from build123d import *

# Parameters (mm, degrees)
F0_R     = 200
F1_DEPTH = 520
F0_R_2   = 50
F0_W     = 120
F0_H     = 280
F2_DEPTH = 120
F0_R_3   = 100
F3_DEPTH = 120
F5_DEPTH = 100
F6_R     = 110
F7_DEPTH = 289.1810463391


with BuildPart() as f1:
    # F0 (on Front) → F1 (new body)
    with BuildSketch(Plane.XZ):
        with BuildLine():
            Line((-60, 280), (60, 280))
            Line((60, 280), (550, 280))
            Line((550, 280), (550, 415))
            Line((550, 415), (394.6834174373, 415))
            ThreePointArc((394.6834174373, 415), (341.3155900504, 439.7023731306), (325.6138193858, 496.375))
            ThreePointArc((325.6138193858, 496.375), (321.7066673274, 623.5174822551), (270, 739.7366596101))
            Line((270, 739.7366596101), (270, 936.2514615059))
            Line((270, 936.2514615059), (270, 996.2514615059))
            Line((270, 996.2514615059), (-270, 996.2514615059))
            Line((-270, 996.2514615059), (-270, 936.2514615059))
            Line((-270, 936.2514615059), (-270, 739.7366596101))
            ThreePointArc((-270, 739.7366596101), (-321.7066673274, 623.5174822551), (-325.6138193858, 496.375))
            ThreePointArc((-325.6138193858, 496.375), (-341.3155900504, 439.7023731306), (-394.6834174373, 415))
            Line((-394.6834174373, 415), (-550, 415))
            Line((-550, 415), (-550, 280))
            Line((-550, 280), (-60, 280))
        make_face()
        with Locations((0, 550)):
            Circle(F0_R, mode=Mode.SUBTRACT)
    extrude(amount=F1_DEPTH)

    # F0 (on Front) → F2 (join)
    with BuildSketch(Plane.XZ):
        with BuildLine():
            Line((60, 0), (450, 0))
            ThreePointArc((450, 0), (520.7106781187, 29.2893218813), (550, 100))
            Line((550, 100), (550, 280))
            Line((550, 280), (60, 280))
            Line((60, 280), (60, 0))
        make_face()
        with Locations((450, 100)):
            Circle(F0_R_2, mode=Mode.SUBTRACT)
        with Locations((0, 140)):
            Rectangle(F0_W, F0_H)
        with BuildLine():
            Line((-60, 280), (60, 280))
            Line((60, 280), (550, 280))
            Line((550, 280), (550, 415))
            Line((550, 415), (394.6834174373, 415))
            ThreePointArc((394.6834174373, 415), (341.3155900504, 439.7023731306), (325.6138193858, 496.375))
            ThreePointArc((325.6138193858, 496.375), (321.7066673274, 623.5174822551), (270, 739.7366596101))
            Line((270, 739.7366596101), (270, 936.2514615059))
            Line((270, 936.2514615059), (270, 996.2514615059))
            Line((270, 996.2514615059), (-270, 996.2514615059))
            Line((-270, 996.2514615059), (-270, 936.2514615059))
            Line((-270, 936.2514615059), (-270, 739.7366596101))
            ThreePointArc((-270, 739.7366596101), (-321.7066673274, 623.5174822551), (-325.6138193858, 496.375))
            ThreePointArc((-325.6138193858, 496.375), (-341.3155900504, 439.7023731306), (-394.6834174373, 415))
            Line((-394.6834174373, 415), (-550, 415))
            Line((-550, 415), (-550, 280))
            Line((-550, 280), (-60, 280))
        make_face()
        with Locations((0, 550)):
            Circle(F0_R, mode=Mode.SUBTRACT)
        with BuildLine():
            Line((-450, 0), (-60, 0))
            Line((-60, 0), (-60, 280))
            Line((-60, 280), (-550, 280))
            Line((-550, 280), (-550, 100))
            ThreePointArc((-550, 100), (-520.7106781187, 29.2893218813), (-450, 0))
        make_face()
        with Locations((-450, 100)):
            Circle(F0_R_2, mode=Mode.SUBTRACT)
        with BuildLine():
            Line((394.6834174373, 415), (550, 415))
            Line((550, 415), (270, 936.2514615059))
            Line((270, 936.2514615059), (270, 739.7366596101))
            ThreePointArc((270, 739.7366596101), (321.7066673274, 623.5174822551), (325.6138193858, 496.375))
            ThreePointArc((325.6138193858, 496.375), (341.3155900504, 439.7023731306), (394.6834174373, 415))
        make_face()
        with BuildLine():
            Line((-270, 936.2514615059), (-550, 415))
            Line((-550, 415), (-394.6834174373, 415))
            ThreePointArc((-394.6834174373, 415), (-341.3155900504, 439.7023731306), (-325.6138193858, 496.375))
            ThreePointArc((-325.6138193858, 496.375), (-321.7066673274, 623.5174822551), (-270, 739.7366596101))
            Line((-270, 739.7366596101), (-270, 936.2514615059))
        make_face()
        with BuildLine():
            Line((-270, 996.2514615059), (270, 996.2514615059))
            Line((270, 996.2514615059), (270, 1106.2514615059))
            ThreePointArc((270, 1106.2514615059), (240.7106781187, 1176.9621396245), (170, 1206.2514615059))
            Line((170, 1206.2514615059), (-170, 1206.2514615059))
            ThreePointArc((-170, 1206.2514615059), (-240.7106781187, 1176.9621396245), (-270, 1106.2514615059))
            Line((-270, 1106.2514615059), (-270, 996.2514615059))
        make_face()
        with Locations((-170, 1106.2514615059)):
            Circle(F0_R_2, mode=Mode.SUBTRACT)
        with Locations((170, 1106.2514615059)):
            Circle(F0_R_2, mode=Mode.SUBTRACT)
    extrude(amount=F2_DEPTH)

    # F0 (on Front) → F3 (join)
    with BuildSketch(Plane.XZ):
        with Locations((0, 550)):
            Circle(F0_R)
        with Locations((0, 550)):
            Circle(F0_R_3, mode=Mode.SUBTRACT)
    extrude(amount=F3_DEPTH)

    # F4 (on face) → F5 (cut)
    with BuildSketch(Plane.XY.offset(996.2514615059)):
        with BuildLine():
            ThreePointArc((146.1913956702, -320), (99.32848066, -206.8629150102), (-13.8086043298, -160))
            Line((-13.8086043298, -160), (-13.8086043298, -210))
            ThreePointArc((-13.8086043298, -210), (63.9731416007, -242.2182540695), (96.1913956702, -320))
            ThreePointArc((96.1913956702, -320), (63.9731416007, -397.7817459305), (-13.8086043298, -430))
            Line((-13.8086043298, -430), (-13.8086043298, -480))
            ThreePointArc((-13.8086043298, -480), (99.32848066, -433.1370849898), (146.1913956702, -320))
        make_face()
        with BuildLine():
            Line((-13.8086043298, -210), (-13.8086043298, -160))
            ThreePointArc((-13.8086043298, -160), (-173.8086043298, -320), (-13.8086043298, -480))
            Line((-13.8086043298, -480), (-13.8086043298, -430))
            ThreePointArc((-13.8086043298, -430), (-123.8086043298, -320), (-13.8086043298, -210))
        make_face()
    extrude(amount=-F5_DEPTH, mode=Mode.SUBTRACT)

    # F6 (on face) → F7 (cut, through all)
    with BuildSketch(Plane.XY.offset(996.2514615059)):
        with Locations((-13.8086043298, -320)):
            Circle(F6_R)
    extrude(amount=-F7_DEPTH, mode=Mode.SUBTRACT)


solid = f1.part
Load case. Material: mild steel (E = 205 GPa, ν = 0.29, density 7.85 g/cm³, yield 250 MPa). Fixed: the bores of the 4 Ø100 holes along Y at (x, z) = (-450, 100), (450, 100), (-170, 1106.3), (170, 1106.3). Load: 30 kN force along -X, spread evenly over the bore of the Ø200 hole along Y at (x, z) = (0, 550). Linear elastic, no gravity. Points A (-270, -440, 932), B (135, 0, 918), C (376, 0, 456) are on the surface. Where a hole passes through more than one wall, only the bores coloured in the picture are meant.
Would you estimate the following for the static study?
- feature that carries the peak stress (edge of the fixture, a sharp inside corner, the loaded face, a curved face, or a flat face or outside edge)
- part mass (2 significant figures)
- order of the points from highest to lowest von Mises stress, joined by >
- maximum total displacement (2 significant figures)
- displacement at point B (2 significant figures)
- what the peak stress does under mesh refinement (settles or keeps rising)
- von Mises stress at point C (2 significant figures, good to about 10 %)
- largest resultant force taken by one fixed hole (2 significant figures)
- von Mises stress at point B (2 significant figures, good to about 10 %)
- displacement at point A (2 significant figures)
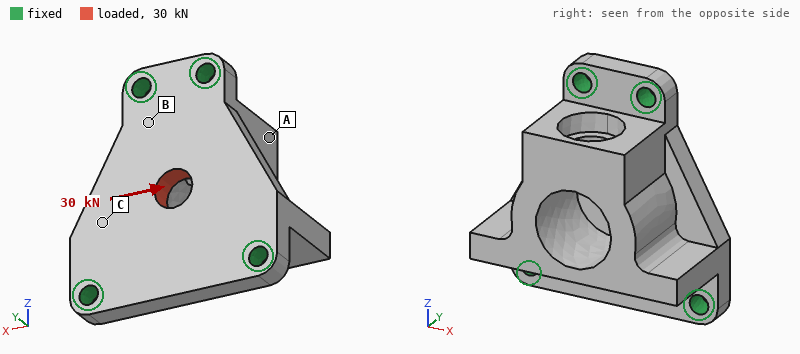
edge of the fixture
2000 kg
B > C > A
1.2 µm
0.45 µm
keeps rising
0.16 MPa
10 kN
0.30 MPa
0.54 µm
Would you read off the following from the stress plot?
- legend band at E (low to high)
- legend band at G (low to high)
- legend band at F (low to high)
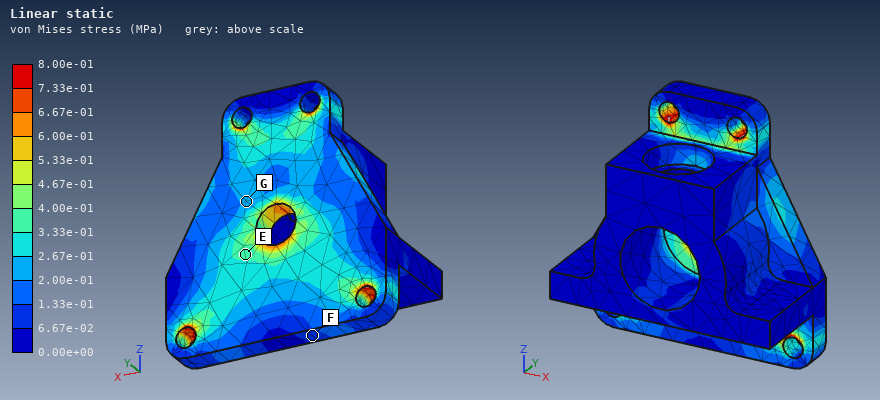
3.33e-01 to 4.00e-01 MPa
2.00e-01 to 2.67e-01 MPa
6.67e-02 to 1.33e-01 MPa
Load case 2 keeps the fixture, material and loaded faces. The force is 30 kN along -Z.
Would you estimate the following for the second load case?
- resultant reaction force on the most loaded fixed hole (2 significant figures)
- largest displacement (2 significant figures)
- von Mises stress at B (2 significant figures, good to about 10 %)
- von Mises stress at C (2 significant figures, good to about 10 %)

8.2 kN
0.94 µm
0.28 MPa
0.091 MPa
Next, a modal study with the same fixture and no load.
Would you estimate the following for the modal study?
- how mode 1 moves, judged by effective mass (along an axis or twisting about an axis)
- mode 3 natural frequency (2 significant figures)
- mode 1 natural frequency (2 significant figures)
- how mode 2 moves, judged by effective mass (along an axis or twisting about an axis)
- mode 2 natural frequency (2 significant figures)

along X
780 Hz
490 Hz
along Y
530 Hz
